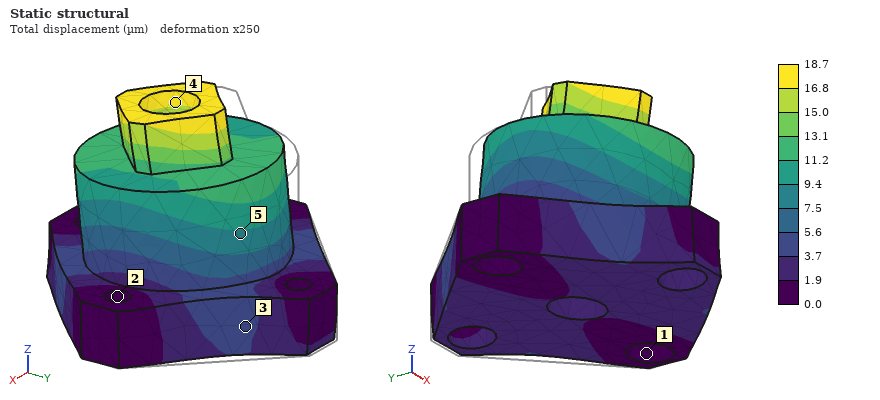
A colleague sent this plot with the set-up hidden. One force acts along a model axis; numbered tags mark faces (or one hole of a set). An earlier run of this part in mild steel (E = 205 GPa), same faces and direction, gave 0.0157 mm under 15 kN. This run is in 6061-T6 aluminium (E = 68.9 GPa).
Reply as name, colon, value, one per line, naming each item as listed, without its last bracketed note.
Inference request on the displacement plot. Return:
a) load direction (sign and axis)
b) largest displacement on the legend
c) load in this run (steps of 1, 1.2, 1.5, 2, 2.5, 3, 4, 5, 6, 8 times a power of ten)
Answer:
load direction: -Y
largest displacement on the legend: 18.7 µm
load in this run: 6 kN
